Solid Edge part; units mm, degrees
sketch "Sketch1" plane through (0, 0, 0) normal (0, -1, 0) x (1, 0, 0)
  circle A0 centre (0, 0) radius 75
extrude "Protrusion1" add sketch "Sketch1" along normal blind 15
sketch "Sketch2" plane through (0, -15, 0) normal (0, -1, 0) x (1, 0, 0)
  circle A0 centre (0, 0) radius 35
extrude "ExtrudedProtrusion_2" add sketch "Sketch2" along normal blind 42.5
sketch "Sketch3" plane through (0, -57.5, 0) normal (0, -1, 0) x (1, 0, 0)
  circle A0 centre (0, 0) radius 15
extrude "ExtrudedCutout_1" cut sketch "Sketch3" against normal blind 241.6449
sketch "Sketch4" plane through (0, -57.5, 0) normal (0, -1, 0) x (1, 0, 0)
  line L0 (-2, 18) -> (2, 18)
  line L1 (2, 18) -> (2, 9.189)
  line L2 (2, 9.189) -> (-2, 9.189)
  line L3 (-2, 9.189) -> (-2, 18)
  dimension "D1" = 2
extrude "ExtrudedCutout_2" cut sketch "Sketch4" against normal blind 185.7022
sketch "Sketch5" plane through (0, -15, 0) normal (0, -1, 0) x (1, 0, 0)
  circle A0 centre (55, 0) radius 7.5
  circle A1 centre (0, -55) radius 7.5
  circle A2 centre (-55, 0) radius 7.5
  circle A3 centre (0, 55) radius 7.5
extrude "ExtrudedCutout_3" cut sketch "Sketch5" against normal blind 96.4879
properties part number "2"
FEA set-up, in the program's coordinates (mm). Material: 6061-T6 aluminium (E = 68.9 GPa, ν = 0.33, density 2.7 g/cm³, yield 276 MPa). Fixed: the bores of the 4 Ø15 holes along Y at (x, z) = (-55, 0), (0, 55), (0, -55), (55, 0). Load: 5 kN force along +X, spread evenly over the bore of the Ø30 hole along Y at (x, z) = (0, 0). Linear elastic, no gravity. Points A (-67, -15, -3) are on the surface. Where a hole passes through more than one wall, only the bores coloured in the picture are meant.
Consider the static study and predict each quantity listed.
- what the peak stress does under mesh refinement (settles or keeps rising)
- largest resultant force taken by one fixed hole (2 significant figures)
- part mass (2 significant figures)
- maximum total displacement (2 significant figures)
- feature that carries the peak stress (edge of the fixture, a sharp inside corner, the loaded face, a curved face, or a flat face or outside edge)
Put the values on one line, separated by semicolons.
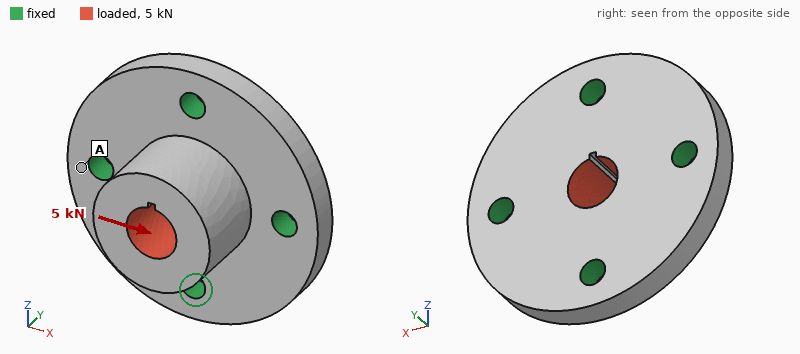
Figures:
keeps rising; 2.0 kN; 1.0 kg; 6.7 µm; edge of the fixture
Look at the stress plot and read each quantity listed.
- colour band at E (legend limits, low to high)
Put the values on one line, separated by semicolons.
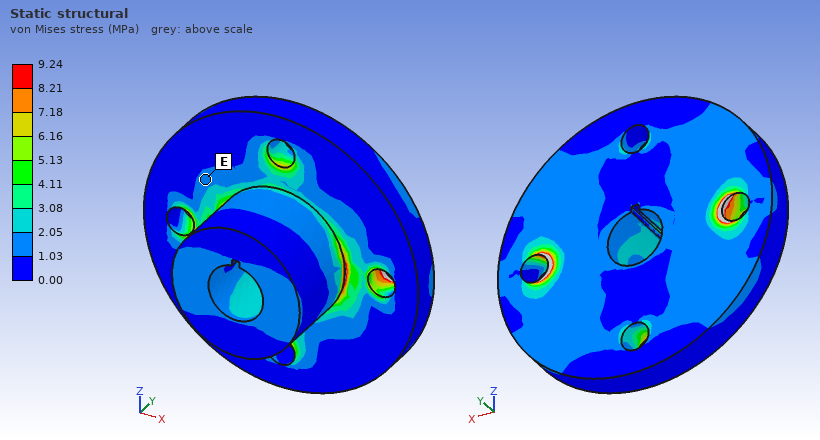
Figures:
1.03 to 2.05 MPa
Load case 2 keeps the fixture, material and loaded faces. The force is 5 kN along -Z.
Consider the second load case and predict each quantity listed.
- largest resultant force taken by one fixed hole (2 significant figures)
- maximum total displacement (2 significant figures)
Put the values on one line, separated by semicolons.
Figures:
2.0 kN; 6.8 µm
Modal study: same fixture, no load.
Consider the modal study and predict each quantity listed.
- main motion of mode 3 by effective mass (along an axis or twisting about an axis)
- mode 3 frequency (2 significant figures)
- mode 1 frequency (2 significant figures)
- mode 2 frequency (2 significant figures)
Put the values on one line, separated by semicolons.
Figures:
along Y; 7700 Hz; 6800 Hz; 6800 Hz
